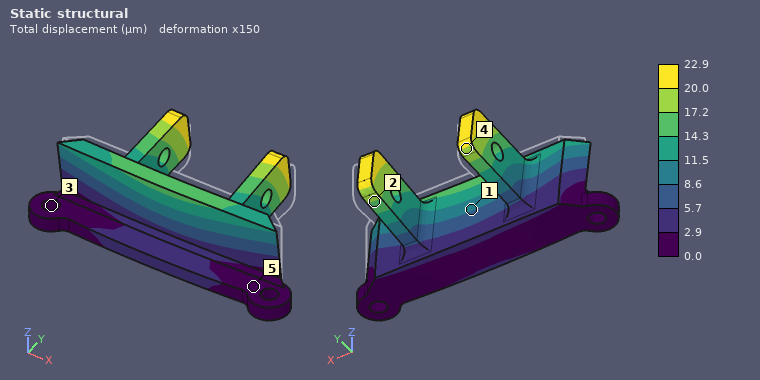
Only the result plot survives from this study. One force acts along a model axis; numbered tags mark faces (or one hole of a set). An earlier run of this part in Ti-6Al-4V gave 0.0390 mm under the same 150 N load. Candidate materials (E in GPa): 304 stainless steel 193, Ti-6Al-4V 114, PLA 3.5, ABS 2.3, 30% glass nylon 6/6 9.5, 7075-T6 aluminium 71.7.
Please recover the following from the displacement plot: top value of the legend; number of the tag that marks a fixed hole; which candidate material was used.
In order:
22.9 µm
3
304 stainless steel
